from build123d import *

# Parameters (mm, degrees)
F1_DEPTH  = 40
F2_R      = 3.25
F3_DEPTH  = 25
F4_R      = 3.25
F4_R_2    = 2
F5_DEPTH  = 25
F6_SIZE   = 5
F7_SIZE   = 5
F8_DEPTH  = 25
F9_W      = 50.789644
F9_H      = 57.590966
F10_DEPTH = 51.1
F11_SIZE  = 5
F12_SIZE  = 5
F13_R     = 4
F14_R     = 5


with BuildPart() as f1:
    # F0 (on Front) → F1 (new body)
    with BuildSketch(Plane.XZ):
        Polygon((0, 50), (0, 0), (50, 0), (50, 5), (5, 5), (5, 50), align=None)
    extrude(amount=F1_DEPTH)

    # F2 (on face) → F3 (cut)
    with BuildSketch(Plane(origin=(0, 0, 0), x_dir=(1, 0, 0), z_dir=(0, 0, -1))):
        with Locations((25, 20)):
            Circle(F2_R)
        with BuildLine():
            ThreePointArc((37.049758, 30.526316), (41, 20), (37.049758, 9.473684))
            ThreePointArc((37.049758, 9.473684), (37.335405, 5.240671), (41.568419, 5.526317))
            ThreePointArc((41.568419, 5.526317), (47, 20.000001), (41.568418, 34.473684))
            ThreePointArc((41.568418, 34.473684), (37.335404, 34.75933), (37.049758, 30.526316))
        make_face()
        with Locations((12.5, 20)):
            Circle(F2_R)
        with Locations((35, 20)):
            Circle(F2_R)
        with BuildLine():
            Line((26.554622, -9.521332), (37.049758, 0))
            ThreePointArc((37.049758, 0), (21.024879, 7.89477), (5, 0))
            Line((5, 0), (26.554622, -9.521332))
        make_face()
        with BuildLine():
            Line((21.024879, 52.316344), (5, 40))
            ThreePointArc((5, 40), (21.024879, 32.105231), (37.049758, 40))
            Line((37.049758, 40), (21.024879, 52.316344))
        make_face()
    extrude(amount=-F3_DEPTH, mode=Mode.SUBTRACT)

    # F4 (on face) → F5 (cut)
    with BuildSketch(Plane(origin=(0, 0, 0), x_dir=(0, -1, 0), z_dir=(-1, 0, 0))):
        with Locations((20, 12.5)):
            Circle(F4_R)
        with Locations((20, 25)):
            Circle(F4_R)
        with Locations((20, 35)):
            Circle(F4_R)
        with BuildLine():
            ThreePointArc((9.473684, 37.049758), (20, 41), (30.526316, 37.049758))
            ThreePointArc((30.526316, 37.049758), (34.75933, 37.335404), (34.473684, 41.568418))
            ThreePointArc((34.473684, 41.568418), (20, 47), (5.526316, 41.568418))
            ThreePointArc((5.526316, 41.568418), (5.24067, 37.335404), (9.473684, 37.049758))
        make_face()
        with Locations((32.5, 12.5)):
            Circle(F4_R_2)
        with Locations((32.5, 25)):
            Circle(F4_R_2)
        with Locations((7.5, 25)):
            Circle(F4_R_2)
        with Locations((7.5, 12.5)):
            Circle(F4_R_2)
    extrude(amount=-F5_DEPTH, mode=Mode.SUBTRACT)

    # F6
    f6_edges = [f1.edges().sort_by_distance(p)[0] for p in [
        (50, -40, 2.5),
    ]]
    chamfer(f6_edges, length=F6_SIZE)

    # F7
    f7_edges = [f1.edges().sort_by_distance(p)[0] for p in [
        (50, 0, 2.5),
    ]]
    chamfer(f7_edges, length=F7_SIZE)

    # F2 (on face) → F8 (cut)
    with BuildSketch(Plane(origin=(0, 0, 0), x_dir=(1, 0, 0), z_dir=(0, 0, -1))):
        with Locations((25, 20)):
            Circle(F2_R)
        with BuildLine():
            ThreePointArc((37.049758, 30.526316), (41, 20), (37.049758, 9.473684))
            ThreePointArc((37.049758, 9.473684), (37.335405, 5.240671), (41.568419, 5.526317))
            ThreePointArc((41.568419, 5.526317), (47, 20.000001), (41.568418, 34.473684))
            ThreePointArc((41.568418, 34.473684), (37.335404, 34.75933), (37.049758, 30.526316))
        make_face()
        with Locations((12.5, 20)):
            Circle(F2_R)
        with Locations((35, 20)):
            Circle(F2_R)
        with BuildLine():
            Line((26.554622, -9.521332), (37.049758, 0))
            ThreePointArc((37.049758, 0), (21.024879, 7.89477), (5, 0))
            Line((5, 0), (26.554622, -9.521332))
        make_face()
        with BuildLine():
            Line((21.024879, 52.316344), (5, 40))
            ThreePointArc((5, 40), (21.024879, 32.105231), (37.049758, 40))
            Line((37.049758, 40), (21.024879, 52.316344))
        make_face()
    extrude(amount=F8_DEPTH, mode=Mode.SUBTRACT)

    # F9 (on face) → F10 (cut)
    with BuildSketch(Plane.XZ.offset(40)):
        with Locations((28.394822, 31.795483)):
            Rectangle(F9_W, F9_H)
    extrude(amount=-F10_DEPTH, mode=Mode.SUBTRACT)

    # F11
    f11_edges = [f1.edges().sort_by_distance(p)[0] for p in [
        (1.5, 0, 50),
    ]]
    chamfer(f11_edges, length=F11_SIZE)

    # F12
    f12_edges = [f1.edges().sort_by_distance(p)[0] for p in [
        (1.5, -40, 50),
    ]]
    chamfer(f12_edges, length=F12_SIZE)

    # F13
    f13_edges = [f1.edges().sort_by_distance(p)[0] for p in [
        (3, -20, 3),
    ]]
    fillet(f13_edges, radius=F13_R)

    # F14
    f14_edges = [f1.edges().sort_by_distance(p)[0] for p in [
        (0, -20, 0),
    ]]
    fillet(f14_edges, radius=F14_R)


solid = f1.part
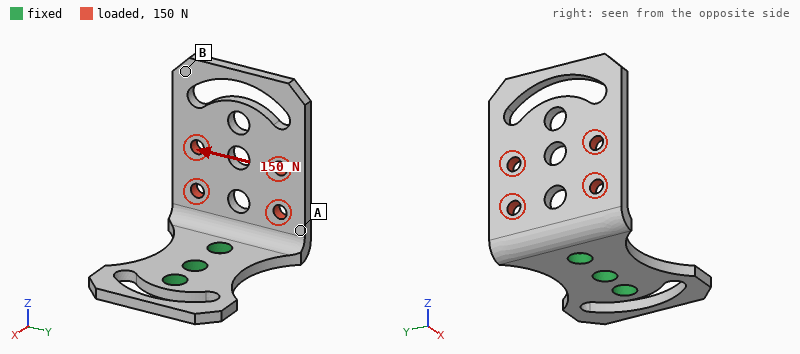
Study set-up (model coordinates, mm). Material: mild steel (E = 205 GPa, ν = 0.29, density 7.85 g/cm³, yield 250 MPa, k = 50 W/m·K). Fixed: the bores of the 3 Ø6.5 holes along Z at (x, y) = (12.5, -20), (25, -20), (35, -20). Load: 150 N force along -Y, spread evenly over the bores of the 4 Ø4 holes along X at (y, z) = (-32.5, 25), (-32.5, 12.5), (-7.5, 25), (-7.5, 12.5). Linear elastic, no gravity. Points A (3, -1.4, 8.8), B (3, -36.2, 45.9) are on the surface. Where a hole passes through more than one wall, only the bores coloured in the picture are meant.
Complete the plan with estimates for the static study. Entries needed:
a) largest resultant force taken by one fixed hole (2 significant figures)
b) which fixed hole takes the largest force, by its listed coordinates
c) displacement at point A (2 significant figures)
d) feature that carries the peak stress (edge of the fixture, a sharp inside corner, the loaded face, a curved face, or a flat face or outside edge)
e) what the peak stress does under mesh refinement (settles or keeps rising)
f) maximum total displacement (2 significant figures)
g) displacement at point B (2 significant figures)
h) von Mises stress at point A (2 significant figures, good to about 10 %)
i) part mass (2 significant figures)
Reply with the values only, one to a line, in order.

190 N
(12.5, -20)
15 µm
edge of the fixture
keeps rising
39 µm
36 µm
9.9 MPa
66 g
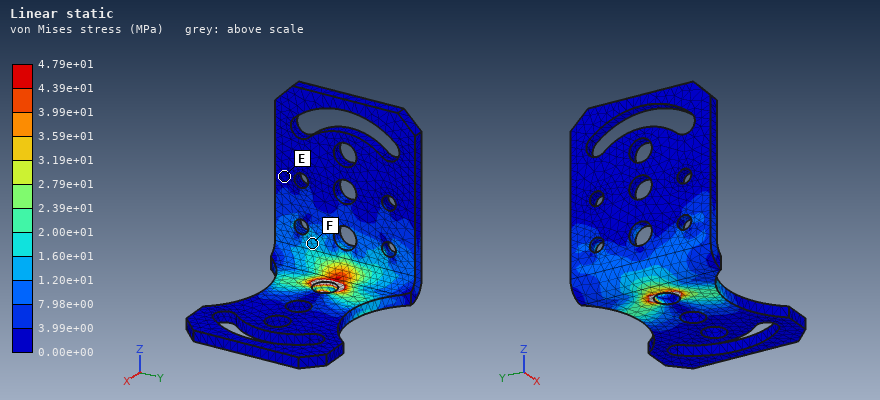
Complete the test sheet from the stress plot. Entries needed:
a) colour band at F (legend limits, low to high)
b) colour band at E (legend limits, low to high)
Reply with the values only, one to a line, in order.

1.20e+01 to 1.60e+01 MPa
0.00e+00 to 3.99e+00 MPa
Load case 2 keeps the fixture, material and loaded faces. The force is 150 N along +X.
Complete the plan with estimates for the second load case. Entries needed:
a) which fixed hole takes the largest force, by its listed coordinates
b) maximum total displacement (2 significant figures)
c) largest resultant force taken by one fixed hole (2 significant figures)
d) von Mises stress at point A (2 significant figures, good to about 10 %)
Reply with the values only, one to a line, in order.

(12.5, -20)
0.11 mm
120 N
26 MPa
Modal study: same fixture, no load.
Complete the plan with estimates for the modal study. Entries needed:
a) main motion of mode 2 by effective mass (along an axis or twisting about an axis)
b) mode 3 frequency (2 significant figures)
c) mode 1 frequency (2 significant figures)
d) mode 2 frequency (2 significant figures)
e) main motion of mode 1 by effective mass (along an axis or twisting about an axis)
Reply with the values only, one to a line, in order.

along Y
2900 Hz
940 Hz
1600 Hz
along X
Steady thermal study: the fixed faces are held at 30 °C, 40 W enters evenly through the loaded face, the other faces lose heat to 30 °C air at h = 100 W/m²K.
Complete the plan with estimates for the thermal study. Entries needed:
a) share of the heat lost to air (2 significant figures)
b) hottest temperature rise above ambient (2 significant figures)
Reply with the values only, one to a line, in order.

64 %
89 K
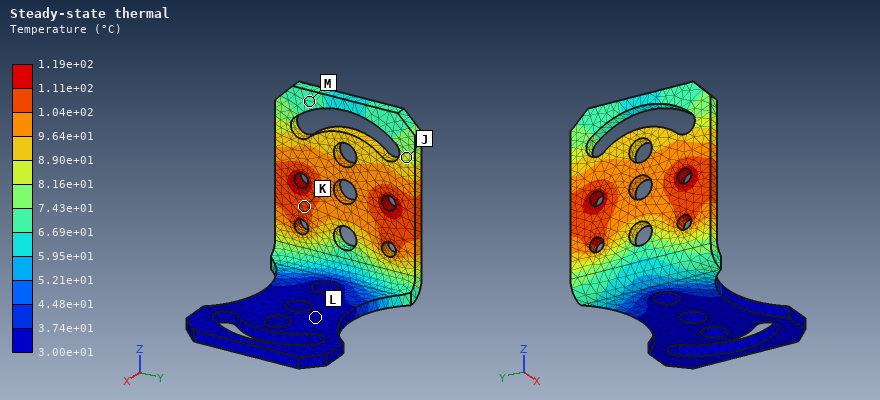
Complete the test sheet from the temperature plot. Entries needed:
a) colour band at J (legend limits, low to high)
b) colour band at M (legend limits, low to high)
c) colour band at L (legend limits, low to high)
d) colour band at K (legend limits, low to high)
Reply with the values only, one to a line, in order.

8.16e+01 to 8.90e+01 °C
6.69e+01 to 7.43e+01 °C
3.00e+01 to 3.74e+01 °C
1.04e+02 to 1.11e+02 °C
